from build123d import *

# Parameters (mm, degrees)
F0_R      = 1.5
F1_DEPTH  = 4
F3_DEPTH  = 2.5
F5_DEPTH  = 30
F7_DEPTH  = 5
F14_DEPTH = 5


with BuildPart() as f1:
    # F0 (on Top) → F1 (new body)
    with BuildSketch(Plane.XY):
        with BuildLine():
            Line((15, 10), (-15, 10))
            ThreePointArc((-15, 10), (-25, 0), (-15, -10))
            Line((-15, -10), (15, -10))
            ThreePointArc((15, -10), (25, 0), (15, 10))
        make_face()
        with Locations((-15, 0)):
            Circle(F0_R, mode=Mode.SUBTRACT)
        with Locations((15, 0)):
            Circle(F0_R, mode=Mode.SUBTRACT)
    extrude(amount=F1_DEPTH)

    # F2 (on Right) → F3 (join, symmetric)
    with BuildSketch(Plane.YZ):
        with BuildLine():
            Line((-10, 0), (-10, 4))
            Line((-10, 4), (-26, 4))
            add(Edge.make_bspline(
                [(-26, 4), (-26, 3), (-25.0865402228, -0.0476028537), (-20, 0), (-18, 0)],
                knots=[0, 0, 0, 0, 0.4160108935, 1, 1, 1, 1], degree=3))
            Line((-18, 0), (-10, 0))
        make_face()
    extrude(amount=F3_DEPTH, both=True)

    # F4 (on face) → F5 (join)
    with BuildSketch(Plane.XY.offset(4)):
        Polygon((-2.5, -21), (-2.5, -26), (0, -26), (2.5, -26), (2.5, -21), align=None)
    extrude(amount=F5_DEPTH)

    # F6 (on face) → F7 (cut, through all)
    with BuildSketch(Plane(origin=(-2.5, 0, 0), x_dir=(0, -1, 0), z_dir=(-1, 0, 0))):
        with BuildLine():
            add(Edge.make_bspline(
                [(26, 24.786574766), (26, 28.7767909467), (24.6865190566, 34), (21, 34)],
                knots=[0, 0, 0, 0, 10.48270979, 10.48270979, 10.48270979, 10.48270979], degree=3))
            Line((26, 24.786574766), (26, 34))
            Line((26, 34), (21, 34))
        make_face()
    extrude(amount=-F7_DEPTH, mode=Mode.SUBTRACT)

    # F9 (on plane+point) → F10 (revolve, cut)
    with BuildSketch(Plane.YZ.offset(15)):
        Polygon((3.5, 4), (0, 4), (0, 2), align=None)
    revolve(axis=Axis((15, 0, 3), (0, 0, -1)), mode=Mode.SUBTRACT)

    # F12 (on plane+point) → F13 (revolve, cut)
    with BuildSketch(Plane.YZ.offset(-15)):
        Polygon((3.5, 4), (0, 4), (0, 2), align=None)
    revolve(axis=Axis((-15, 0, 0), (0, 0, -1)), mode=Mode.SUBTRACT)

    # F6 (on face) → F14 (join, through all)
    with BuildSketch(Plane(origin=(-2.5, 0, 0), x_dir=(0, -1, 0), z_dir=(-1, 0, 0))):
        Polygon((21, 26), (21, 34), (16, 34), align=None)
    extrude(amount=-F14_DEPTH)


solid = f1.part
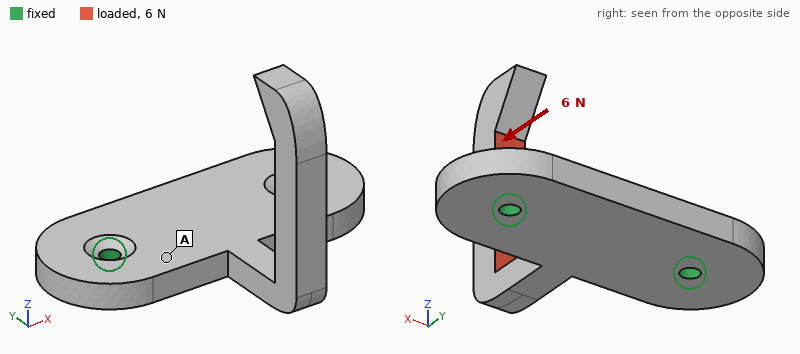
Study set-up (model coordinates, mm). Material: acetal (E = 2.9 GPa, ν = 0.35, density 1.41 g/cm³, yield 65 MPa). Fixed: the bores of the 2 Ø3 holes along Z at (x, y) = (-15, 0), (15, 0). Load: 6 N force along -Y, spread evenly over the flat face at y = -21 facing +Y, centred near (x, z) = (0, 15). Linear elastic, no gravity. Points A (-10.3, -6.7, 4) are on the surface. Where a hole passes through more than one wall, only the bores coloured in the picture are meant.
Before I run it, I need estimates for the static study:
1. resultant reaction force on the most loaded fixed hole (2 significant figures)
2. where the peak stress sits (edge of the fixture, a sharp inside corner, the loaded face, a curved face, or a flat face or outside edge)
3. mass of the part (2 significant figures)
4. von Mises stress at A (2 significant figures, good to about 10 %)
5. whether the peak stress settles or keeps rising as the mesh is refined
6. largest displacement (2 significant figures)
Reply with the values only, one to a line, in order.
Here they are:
3.0 N
a sharp inside corner
6.6 g
0.86 MPa
keeps rising
0.69 mm
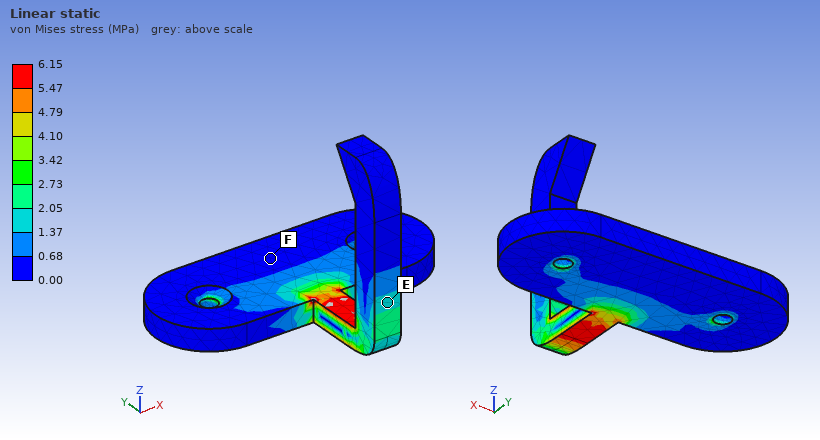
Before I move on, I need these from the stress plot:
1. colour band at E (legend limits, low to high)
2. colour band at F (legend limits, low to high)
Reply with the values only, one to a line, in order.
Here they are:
1.37 to 2.05 MPa
0.00 to 0.68 MPa
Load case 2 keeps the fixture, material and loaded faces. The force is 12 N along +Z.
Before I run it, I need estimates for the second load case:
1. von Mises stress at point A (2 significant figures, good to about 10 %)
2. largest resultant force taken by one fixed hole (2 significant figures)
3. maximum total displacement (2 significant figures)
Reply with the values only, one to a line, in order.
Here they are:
2.2 MPa
7.1 N
0.70 mm
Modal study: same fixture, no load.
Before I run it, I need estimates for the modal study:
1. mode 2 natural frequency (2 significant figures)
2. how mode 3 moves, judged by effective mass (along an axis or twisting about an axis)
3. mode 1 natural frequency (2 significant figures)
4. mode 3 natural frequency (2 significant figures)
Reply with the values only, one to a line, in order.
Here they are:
430 Hz
along Z
410 Hz
1200 Hz
